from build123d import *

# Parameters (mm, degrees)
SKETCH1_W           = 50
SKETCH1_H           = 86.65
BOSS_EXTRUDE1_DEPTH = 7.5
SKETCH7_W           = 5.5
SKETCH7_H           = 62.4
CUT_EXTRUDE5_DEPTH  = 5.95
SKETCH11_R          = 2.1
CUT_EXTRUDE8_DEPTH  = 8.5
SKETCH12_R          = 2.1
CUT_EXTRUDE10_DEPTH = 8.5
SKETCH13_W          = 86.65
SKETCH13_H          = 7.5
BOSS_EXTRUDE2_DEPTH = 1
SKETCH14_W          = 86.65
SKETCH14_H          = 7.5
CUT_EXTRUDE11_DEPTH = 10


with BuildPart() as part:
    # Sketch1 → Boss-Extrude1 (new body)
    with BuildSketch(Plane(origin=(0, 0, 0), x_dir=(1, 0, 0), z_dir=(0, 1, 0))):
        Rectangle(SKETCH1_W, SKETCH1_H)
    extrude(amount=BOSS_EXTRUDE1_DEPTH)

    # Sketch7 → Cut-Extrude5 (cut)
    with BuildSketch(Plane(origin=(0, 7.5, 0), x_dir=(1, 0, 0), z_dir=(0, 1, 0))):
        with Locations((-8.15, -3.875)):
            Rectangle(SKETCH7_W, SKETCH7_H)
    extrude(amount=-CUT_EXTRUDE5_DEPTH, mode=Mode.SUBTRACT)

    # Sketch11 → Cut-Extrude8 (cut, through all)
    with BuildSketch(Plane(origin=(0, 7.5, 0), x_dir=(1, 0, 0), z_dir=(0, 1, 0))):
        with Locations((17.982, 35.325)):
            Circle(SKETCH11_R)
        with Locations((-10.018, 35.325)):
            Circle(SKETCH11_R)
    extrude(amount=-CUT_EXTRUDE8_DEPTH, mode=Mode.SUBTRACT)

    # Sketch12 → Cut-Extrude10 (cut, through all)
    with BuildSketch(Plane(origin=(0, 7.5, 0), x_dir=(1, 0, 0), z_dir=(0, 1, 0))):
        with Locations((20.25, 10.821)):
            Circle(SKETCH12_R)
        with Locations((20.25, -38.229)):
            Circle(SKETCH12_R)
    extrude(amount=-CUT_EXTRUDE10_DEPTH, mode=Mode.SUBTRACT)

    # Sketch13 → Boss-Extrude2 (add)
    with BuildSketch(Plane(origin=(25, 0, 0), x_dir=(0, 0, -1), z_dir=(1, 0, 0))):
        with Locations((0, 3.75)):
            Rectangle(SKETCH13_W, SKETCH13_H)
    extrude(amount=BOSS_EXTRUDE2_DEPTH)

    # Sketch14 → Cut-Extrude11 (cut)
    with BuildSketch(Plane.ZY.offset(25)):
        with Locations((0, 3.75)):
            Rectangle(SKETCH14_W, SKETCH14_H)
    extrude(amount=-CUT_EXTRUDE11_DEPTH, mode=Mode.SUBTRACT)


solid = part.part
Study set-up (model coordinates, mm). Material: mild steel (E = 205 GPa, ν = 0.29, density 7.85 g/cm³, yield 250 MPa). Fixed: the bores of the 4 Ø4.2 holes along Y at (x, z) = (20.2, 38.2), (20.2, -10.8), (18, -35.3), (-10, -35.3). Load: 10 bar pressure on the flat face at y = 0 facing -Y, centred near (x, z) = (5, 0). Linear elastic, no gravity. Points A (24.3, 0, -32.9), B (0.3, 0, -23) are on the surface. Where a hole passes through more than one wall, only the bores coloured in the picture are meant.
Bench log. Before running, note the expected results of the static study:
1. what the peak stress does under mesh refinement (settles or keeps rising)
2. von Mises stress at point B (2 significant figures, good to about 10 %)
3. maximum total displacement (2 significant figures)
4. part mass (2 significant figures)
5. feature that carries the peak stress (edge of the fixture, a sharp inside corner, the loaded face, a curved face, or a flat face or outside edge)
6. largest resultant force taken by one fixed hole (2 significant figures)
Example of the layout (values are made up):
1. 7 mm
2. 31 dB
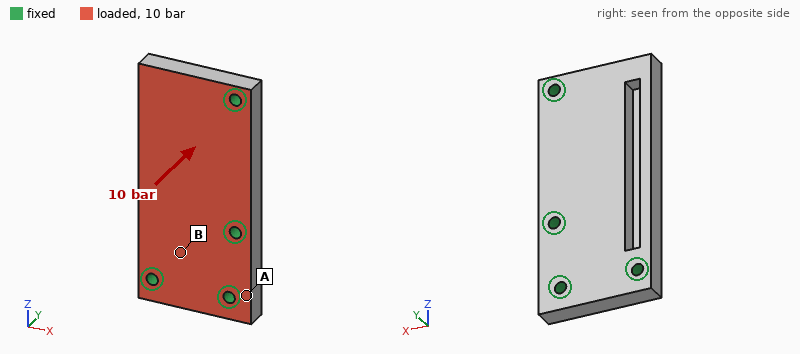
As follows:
1. keeps rising
2. 29 MPa
3. 41 µm
4. 190 g
5. edge of the fixture
6. 1.2 kN
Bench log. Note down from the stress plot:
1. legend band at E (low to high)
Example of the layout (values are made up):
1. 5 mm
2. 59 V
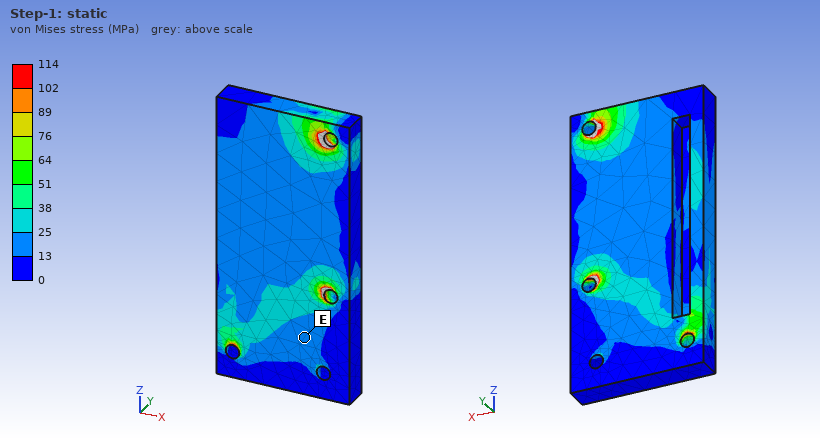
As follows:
1. 13 to 25 MPa
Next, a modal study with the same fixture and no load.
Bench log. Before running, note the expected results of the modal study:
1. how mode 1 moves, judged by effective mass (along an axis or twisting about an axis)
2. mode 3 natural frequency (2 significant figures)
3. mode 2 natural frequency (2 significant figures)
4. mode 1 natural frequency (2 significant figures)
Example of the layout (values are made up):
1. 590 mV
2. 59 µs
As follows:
1. along Y
2. 12 kHz
3. 9900 Hz
4. 4800 Hz
